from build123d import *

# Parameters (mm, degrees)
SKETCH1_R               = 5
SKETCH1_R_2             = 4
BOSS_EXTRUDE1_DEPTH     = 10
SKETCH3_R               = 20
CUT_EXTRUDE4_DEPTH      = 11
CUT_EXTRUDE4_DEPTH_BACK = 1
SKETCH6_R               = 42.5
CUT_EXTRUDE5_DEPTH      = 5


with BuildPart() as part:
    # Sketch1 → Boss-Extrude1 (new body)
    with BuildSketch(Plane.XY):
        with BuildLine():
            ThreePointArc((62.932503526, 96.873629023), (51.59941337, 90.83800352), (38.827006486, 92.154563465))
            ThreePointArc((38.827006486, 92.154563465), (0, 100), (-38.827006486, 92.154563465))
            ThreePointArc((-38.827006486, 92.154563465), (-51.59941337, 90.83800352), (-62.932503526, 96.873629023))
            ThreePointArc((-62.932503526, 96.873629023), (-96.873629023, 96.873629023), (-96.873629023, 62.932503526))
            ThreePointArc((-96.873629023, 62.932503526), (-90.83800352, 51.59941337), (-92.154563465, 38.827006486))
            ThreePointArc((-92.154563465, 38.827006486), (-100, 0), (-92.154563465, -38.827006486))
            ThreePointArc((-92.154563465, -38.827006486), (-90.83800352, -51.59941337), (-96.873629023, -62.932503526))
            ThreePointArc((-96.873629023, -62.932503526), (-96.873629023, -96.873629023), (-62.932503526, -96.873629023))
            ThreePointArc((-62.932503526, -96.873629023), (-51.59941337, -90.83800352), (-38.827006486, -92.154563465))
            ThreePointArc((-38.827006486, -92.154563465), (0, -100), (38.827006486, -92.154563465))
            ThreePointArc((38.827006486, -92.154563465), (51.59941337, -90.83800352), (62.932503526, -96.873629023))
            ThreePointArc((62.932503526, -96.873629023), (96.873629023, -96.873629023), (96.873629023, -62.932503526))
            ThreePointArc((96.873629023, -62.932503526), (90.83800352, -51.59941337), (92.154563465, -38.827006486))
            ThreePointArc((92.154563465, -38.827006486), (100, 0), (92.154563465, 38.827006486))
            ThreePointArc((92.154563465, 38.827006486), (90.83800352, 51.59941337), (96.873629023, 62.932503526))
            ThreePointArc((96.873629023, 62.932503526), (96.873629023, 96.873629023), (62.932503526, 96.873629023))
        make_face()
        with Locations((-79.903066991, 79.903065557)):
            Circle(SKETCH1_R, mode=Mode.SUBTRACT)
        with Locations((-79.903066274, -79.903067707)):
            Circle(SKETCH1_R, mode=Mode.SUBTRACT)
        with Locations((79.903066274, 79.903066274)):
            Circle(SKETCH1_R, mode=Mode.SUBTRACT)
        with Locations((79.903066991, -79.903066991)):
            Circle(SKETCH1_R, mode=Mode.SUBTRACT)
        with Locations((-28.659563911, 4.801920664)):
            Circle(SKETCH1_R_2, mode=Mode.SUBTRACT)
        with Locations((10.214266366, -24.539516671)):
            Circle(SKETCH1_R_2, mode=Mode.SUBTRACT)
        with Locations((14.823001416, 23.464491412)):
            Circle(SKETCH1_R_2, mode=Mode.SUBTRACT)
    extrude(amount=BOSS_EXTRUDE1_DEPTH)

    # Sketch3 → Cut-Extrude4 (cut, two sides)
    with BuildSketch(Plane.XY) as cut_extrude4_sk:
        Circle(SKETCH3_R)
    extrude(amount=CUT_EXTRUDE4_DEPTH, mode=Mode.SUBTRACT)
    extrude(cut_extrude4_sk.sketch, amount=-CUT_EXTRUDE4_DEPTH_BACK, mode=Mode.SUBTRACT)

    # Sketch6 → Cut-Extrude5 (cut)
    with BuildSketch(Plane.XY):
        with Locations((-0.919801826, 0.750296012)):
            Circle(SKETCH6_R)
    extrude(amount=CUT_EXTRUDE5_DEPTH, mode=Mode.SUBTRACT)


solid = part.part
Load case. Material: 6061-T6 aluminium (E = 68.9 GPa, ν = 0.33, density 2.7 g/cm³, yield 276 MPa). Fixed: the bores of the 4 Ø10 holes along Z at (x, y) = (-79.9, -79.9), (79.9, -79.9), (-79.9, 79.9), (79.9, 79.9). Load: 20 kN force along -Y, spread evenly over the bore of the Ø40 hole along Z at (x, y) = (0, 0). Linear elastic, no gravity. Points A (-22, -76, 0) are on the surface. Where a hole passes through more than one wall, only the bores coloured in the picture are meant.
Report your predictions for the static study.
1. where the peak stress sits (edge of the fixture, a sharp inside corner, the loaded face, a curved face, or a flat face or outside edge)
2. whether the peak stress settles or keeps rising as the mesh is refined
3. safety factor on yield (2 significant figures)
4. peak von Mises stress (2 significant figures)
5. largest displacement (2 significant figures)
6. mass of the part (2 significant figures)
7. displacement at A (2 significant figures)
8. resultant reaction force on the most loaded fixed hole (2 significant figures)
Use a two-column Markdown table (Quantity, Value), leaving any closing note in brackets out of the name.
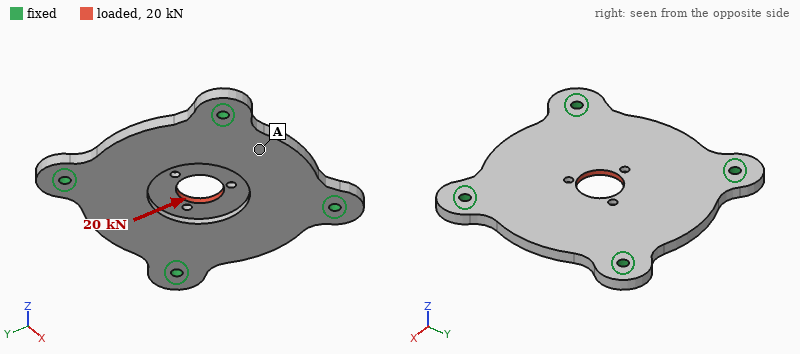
| Quantity | Value |
|---|---|
| where the peak stress sits | a curved face |
| whether the peak stress settles or keeps rising as the mesh is refined | settles |
| safety factor on yield | 2.4 |
| peak von Mises stress | 120 MPa |
| largest displacement | 44 µm |
| mass of the part | 920 g |
| displacement at A | 17 µm |
| resultant reaction force on the most loaded fixed hole | 5.8 kN |
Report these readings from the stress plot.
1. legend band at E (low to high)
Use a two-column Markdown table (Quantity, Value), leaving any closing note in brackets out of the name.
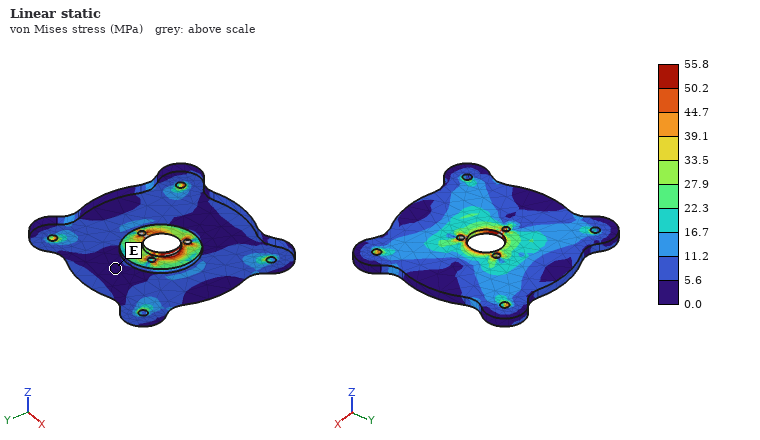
| Quantity | Value |
|---|---|
| legend band at E | 0.0 to 5.6 MPa |
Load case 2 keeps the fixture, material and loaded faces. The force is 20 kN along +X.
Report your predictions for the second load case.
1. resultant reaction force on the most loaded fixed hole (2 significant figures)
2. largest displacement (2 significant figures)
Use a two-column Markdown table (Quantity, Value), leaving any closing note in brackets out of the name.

| Quantity | Value |
|---|---|
| resultant reaction force on the most loaded fixed hole | 5.7 kN |
| largest displacement | 41 µm |
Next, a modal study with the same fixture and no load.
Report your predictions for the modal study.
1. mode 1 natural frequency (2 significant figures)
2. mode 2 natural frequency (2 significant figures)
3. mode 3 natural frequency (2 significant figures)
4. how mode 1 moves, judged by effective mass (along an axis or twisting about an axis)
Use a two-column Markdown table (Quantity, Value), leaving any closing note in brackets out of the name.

| Quantity | Value |
|---|---|
| mode 1 natural frequency | 1400 Hz |
| mode 2 natural frequency | 2100 Hz |
| mode 3 natural frequency | 2100 Hz |
| how mode 1 moves, judged by effective mass | along Z |
